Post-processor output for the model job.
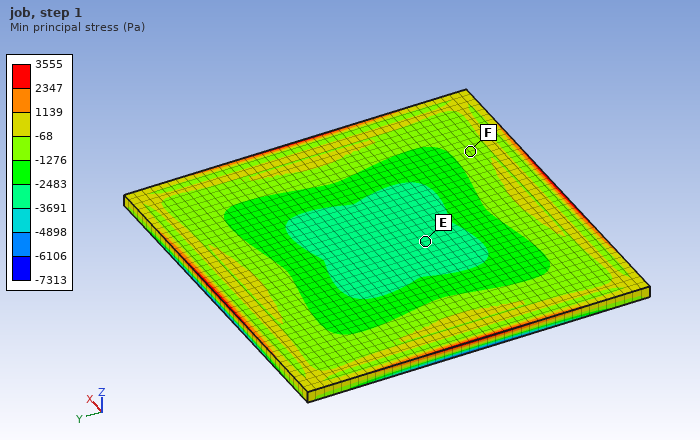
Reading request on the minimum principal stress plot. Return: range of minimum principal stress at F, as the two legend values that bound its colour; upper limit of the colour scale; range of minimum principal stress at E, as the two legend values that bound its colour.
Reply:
-1276 to -68 Pa
3555 Pa
-3691 to -2483 Pa
